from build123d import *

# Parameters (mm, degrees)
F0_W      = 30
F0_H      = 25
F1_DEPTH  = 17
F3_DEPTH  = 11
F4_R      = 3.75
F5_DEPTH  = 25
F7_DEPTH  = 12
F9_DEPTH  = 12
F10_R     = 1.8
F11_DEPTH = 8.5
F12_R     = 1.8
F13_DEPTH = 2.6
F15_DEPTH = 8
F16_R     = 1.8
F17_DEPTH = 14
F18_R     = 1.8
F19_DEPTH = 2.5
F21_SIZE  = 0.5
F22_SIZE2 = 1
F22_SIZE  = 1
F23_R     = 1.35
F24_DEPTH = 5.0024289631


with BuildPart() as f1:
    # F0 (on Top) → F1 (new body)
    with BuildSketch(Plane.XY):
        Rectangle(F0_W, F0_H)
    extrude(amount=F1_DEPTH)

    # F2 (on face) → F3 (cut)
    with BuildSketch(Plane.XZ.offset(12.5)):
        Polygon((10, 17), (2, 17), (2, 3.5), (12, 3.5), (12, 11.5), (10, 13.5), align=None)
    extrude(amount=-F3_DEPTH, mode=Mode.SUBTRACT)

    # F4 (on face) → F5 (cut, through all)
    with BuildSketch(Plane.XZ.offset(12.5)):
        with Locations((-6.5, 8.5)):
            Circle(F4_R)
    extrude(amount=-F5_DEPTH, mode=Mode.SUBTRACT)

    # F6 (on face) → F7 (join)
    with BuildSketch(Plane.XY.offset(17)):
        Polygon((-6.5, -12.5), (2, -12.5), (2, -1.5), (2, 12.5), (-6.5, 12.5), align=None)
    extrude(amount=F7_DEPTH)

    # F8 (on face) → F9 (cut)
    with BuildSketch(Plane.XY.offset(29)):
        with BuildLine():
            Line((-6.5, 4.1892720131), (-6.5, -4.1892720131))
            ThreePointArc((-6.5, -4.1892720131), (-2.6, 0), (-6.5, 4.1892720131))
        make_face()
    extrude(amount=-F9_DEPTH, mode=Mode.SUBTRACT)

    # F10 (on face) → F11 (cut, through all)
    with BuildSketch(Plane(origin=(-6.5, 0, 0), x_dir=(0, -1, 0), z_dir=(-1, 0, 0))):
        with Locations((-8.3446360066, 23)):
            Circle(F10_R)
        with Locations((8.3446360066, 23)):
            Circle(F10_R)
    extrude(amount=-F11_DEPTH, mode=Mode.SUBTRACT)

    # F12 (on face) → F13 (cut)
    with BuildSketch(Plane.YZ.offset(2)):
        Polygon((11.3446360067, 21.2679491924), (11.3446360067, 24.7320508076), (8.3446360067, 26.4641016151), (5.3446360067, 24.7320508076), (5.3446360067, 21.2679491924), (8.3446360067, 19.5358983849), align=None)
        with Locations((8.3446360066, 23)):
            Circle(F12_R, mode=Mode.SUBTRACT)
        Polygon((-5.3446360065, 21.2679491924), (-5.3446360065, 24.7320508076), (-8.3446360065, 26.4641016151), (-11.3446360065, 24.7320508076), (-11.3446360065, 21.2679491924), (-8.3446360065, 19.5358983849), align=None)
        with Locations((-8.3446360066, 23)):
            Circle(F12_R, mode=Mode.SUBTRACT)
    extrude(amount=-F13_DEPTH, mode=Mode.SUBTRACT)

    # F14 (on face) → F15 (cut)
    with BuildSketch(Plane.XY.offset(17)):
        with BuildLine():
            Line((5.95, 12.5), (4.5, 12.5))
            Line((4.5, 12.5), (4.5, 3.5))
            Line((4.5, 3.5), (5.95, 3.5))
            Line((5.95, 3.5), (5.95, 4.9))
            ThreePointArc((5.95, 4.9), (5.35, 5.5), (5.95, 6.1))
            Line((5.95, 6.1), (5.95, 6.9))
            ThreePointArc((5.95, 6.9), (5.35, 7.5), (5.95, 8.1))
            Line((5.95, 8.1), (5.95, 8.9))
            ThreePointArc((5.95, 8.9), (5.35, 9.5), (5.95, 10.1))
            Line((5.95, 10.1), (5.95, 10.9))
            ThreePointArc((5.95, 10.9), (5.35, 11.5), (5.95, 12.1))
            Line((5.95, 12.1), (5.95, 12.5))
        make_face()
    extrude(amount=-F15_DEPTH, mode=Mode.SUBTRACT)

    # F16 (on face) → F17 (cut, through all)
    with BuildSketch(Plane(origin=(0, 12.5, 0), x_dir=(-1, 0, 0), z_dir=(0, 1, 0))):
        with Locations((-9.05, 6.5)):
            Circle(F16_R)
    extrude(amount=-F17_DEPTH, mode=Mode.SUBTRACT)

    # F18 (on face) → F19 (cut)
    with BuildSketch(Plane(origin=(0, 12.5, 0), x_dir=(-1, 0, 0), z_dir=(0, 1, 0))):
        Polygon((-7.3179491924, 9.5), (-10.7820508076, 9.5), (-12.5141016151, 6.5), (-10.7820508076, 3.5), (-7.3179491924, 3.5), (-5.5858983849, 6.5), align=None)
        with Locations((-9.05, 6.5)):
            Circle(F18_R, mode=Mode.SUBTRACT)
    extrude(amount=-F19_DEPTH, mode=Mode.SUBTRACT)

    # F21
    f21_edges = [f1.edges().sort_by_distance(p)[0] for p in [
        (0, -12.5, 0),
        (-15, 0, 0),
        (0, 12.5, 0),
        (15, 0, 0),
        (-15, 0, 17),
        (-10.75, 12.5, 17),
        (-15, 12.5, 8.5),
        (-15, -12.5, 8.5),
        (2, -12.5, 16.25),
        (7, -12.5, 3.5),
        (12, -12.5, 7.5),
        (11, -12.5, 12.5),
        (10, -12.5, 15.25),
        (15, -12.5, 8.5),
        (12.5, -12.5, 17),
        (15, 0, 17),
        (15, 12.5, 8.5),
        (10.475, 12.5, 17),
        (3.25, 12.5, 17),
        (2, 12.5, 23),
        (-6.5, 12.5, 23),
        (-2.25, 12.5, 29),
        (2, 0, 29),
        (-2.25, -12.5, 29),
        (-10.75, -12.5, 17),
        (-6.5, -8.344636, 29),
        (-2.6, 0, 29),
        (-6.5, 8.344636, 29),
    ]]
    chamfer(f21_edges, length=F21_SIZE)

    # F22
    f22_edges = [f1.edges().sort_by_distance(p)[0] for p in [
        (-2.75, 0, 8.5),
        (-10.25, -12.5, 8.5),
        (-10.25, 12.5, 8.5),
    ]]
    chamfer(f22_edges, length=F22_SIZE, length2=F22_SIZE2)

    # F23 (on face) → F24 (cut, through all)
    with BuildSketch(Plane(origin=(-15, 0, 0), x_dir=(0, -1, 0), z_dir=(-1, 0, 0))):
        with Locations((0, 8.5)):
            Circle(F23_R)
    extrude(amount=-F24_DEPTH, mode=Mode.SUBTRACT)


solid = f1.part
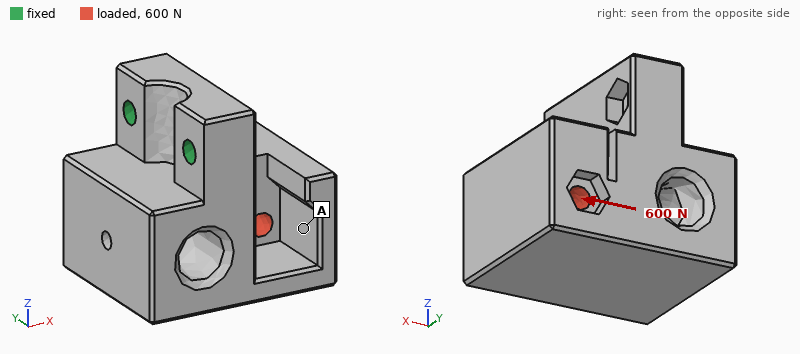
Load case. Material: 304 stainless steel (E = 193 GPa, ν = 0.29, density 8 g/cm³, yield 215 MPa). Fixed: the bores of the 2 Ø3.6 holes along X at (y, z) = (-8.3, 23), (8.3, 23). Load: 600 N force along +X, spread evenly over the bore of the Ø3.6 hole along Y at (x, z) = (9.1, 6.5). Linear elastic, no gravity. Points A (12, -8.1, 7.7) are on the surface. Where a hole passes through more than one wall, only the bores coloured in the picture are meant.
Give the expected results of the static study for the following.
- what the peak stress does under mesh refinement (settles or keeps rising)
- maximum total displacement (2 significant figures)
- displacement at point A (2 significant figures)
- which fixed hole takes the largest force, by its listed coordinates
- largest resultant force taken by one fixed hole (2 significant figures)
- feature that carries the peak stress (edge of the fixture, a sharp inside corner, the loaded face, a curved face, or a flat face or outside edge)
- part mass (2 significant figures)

keeps rising
15 µm
11 µm
(8.3, 23)
430 N
edge of the fixture
95 g
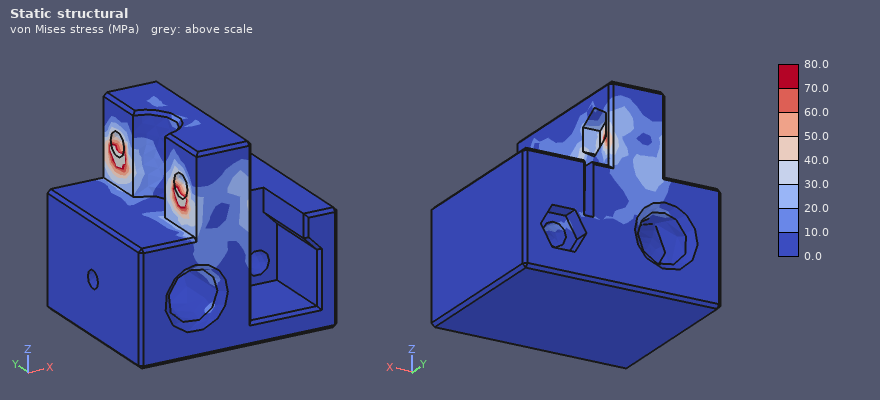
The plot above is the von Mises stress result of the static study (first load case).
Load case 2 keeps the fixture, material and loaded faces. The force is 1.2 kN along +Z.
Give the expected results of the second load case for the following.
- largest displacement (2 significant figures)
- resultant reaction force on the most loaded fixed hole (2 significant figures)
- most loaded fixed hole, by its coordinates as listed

28 µm
900 N
(8.3, 23)
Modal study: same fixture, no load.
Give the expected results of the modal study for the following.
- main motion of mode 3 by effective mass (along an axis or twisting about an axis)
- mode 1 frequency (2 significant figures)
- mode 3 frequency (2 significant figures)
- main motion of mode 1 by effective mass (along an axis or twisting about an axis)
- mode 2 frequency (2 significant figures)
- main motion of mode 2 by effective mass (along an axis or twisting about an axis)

along Y
4300 Hz
13 kHz
along X
10 kHz
along Y
